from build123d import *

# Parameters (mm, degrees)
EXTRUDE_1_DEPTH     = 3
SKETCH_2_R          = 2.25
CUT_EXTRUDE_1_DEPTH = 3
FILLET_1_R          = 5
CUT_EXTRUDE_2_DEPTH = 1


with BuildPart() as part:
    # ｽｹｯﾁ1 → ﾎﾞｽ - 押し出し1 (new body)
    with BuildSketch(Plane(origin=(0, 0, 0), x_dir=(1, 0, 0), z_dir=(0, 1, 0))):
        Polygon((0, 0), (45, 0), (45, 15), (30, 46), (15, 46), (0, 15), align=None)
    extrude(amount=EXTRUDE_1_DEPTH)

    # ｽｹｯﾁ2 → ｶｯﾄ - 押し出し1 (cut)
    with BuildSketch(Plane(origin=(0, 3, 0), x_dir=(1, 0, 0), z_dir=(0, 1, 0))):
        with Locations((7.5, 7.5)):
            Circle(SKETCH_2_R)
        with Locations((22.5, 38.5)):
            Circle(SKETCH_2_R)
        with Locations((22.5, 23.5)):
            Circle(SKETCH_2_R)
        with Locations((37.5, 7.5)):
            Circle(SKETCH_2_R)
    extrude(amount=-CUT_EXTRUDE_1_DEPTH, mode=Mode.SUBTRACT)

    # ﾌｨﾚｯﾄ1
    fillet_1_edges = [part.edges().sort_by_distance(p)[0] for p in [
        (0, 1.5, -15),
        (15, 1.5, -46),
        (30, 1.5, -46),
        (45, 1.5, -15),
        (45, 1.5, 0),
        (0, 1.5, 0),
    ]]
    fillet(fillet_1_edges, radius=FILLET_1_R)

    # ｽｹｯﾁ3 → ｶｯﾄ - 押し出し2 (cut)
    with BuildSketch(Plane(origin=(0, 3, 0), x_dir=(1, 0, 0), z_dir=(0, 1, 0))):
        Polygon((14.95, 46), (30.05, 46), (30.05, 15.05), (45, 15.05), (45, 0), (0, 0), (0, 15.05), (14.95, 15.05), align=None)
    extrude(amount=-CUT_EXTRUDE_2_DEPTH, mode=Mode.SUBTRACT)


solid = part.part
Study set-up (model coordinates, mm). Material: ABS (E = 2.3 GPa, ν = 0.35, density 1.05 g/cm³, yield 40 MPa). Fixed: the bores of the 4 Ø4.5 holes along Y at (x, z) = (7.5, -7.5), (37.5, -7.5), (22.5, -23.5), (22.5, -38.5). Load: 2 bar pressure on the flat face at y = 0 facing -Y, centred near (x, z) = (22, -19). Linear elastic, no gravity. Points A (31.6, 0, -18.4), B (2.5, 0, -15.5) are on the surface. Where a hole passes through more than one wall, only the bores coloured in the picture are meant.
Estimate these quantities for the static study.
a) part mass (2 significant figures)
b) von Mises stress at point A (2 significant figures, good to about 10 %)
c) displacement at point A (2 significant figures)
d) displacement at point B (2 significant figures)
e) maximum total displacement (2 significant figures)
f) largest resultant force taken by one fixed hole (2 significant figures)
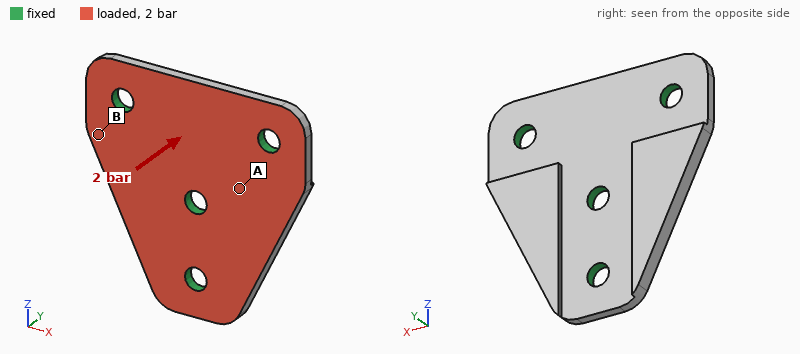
3.7 g
7.0 MPa
0.080 mm
0.14 mm
0.27 mm
82 N
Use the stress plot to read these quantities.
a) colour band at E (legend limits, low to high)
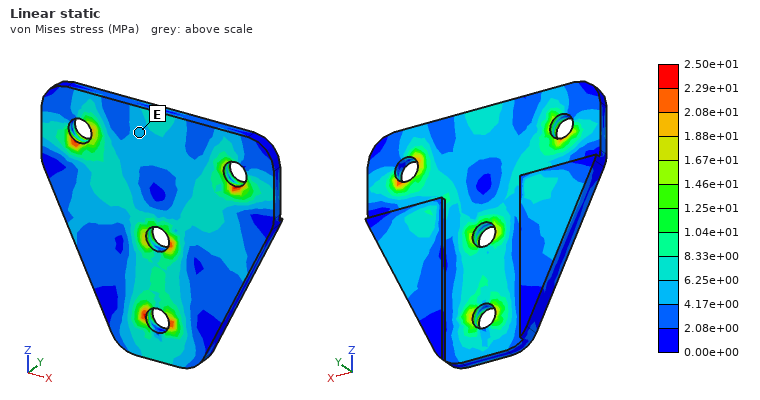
4.17e+00 to 6.25e+00 MPa
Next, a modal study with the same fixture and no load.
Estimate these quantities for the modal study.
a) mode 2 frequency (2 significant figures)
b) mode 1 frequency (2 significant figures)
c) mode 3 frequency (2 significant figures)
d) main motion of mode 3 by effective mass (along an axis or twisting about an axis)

3100 Hz
3100 Hz
4200 Hz
along Y
